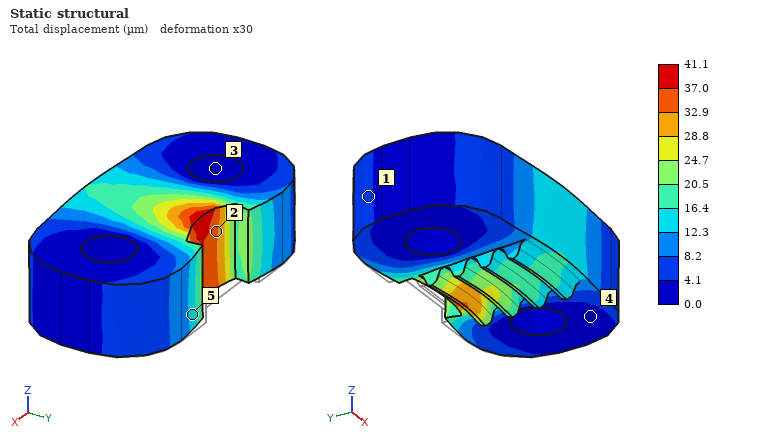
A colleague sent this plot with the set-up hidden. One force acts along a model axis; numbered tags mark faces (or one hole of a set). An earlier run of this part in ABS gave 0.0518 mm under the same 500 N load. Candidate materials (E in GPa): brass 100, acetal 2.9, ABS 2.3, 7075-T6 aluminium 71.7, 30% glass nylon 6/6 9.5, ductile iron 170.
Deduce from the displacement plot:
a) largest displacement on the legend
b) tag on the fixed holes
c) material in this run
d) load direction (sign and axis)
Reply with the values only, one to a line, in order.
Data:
41.1 µm
3
acetal
-Y
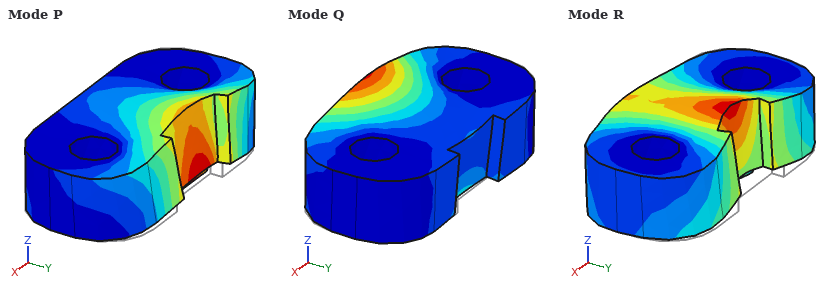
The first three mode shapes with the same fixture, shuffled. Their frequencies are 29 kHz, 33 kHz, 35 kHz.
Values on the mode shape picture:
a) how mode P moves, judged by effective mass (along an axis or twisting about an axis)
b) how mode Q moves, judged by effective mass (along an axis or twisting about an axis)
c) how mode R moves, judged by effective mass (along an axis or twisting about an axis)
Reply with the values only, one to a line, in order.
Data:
along Z
along Z
along Y
